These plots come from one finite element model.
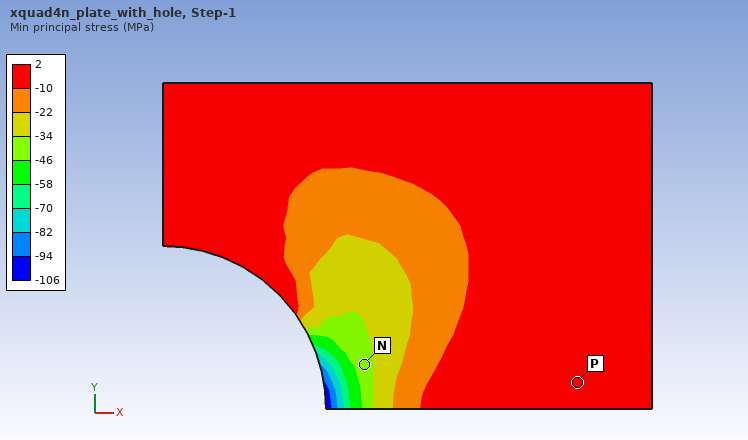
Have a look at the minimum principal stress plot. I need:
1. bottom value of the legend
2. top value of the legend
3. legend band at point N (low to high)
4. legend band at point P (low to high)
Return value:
-106 MPa
2 MPa
-46 to -34 MPa
-10 to 2 MPa
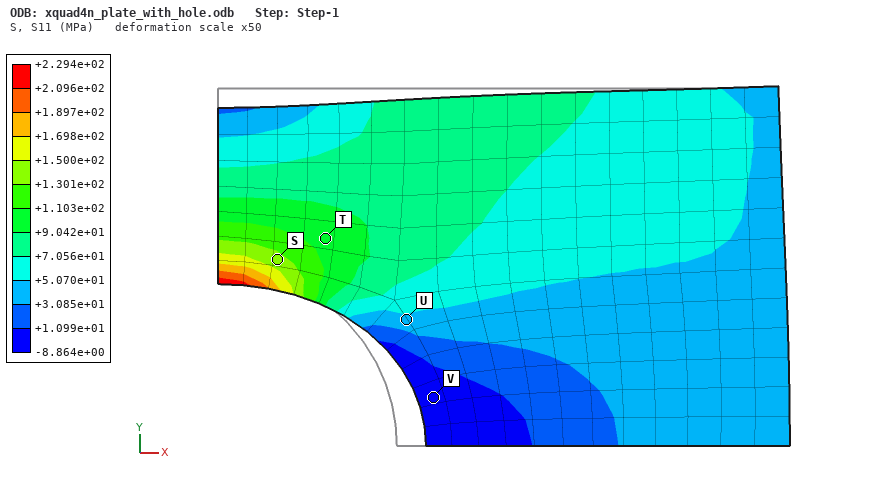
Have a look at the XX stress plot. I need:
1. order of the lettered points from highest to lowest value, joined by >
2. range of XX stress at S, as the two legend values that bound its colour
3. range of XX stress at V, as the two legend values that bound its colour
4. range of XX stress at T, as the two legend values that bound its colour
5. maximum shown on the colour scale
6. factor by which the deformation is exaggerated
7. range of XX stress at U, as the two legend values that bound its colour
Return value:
S > T > U > V
+1.301e+02 to +1.500e+02 MPa
-8.864e+00 to +1.099e+01 MPa
+9.042e+01 to +1.103e+02 MPa
+2.294e+02 MPa
50
+3.085e+01 to +5.070e+01 MPa
